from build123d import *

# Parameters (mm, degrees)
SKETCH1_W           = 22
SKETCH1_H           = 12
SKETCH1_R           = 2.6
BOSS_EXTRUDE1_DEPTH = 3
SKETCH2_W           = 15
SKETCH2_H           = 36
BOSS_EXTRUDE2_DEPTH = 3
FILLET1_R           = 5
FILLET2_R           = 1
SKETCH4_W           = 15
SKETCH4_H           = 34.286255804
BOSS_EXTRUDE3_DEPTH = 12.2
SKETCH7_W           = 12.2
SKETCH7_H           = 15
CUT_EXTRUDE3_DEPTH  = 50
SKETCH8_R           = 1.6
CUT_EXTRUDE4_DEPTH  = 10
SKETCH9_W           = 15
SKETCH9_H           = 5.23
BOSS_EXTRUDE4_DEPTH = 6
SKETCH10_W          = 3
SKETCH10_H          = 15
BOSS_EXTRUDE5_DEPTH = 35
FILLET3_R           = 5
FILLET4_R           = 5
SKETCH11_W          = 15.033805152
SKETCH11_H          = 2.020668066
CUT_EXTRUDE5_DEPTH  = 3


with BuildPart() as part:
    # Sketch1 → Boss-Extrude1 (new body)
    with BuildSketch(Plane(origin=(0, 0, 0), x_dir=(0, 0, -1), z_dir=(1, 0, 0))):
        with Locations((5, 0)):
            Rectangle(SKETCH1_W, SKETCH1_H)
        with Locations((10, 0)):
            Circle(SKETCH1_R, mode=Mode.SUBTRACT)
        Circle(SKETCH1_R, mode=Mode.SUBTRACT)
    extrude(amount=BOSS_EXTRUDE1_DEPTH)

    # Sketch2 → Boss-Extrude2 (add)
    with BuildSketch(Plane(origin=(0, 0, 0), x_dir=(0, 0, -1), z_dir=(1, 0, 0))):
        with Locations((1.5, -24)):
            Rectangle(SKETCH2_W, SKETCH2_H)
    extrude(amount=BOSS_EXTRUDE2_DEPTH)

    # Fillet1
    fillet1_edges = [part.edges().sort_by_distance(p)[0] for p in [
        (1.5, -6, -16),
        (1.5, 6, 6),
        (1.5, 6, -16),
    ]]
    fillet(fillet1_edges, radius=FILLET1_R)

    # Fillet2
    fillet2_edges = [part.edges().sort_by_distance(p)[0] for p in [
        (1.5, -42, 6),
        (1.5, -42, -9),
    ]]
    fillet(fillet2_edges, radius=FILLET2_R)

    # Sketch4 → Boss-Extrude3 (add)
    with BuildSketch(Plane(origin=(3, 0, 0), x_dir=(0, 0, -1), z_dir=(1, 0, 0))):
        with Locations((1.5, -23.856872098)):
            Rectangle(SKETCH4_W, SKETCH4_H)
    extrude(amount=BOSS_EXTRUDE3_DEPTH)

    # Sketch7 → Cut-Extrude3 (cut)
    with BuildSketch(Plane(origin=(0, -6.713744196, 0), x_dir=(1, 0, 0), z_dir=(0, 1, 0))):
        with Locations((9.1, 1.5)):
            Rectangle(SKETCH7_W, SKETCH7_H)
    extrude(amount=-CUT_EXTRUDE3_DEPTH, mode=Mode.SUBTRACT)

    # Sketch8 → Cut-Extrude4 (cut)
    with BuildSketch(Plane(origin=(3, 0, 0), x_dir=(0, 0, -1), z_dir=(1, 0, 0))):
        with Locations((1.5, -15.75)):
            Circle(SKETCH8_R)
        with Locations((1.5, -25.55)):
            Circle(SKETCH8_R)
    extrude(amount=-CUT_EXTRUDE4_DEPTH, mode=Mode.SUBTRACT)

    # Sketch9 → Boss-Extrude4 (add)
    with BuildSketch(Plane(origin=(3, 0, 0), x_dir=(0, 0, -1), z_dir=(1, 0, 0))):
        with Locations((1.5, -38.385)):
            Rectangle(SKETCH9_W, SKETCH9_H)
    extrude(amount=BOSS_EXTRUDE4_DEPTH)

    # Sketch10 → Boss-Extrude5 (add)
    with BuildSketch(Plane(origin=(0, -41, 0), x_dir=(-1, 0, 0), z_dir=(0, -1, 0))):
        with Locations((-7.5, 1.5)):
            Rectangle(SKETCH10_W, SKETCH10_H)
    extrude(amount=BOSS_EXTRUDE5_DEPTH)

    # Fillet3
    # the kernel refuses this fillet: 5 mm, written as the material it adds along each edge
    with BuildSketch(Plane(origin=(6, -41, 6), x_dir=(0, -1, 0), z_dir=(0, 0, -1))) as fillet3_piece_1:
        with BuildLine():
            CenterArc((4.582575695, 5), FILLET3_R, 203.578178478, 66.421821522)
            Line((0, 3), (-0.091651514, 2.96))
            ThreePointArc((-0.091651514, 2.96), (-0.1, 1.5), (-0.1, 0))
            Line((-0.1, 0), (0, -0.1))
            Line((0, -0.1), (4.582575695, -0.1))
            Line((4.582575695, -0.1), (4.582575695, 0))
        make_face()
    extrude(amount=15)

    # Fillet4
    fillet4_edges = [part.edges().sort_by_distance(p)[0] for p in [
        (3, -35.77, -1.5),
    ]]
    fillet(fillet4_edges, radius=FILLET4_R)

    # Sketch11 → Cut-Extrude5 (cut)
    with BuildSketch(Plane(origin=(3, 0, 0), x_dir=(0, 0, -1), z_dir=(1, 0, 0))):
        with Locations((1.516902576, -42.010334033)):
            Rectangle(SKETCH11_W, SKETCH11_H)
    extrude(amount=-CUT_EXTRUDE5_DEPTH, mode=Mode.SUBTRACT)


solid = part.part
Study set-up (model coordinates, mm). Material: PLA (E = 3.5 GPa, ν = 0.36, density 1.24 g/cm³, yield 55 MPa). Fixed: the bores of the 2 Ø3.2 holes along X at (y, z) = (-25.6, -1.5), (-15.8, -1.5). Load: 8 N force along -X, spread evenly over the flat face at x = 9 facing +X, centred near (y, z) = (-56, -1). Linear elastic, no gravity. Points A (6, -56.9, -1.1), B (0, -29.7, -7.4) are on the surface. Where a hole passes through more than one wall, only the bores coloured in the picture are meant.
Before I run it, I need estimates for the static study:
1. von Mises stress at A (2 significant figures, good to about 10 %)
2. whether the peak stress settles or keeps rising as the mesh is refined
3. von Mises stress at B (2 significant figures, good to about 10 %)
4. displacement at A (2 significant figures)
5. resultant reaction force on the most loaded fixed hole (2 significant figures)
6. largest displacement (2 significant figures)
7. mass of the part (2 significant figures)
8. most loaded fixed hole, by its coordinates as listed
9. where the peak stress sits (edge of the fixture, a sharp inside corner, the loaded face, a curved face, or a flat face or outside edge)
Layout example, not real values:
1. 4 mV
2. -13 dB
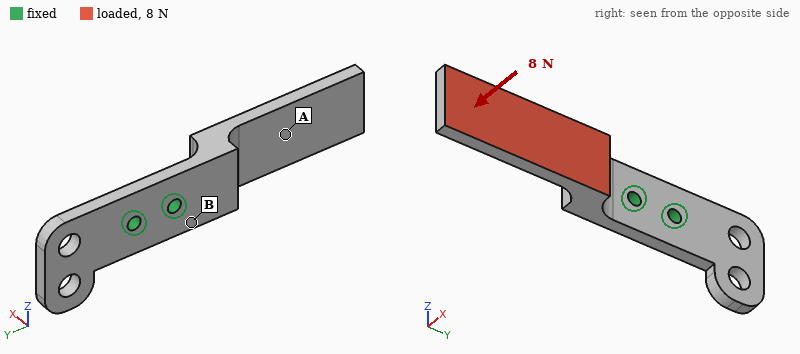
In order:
1. 1.6 MPa
2. keeps rising
3. 7.8 MPa
4. 0.47 mm
5. 15 N
6. 0.95 mm
7. 5.4 g
8. (-25.6, -1.5)
9. edge of the fixture
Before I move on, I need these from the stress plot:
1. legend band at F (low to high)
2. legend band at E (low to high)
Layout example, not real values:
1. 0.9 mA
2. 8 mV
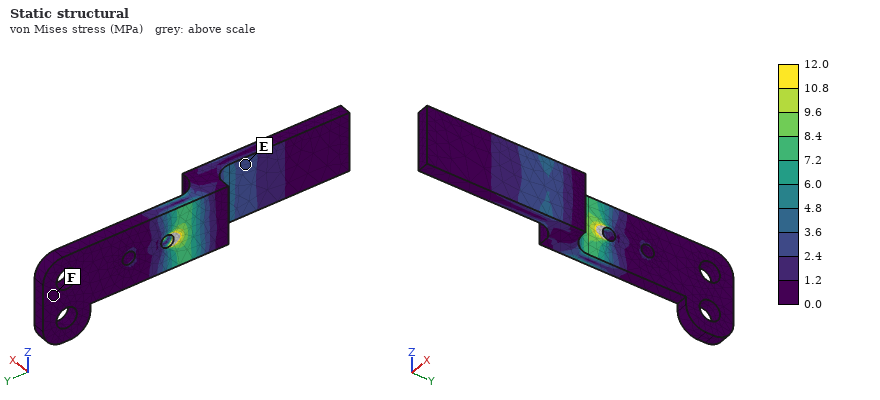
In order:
1. 0.0 to 1.2 MPa
2. 2.4 to 3.6 MPa
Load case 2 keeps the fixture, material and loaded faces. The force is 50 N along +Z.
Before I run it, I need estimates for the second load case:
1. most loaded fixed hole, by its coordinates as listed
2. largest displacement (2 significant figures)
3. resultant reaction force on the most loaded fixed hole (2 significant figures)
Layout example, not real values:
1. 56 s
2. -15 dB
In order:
1. (-25.6, -1.5)
2. 0.63 mm
3. 150 N
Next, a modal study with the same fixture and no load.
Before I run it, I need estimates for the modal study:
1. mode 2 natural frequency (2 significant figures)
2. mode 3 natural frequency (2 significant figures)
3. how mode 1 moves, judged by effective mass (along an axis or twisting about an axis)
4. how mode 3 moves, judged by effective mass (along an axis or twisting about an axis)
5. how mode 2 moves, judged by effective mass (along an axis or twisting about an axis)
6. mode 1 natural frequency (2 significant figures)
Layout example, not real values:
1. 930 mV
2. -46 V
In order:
1. 1200 Hz
2. 1600 Hz
3. along X
4. along X
5. along Z
6. 380 Hz
